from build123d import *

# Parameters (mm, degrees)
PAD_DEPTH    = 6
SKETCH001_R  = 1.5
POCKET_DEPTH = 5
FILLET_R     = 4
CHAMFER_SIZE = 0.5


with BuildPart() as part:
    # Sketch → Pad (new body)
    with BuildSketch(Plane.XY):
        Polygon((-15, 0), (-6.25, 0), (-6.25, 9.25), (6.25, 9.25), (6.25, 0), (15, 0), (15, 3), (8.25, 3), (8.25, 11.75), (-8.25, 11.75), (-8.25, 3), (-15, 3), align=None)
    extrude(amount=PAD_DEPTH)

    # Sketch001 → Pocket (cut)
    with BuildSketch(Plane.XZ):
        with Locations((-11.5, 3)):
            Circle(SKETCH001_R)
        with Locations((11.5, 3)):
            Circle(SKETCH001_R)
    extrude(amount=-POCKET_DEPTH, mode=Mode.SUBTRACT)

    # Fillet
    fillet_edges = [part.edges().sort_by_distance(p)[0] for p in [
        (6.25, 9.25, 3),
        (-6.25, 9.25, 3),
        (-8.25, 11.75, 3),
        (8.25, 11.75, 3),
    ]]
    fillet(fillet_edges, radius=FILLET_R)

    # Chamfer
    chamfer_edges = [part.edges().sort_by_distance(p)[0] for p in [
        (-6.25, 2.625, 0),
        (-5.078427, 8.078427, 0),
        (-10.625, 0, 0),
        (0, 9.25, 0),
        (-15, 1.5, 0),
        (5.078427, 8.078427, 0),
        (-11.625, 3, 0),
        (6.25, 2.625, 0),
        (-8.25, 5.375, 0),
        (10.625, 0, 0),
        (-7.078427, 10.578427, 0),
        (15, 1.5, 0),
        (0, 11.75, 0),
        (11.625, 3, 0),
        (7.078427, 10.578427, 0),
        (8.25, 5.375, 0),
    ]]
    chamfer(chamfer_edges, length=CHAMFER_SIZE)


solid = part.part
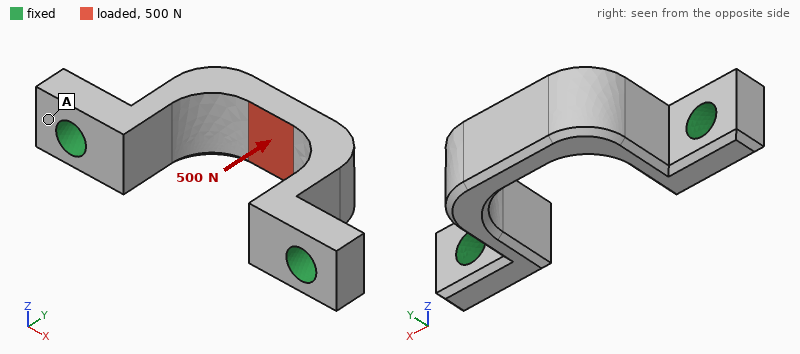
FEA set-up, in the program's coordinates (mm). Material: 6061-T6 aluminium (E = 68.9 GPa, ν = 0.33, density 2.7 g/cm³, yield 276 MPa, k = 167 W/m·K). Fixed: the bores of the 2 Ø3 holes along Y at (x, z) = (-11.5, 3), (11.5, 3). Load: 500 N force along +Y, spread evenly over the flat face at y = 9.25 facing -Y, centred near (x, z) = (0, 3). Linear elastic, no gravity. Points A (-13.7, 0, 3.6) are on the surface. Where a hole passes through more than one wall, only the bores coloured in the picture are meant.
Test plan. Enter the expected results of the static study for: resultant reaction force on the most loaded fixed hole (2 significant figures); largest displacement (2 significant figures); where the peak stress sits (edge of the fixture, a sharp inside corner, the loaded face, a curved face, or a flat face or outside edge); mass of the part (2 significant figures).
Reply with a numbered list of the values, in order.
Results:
1. 290 N
2. 21 µm
3. a flat face or outside edge
4. 1.8 g
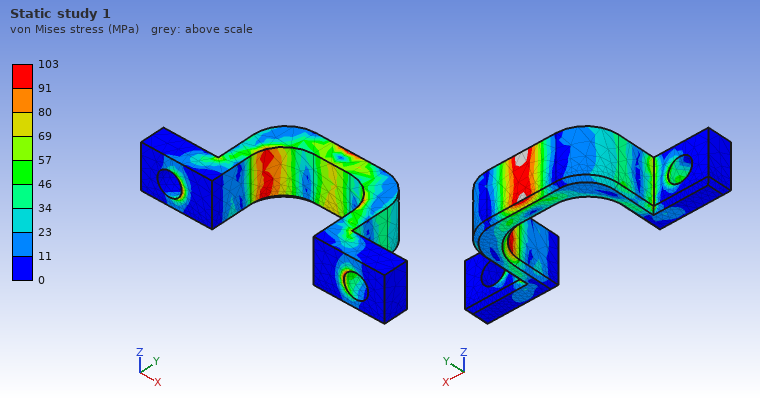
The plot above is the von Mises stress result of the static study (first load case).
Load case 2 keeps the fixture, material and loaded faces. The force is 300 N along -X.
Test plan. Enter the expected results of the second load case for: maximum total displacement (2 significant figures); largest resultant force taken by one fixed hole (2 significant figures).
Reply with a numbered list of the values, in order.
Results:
1. 25 µm
2. 170 N
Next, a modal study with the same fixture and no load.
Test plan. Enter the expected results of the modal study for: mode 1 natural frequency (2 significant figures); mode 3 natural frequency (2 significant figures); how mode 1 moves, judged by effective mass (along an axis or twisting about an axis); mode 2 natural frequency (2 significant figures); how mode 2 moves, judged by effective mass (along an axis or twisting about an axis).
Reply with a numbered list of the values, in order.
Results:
1. 14 kHz
2. 27 kHz
3. along Z
4. 21 kHz
5. along X
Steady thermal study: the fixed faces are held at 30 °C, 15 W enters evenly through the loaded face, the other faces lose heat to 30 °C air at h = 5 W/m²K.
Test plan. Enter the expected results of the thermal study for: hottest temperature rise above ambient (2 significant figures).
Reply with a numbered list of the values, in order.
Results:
1. 49 K
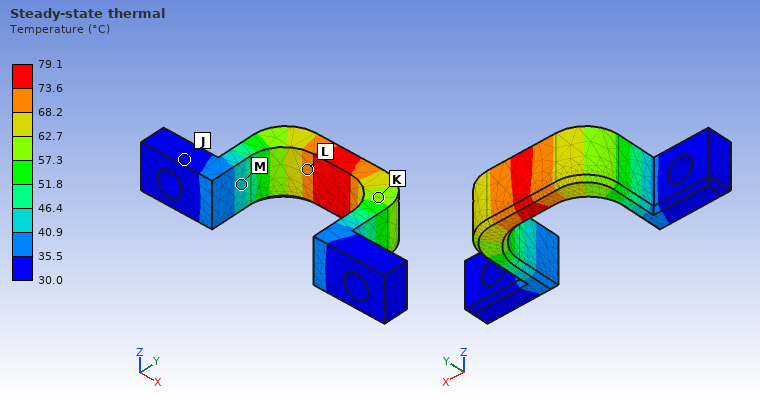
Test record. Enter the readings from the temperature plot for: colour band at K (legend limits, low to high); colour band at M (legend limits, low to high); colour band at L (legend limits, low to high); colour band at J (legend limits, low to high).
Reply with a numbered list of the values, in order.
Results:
1. 57.3 to 62.7 °C
2. 40.9 to 46.4 °C
3. 68.2 to 73.6 °C
4. 30.0 to 35.5 °C
